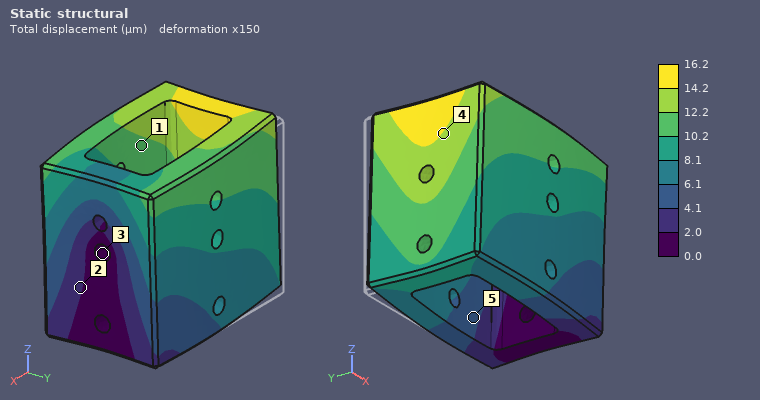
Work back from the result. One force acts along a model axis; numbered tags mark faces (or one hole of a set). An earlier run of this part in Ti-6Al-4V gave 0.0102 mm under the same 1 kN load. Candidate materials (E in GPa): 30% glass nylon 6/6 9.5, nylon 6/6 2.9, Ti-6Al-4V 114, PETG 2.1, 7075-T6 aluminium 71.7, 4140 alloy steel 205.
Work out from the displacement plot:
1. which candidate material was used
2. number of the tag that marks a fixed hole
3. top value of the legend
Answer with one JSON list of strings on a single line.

["7075-T6 aluminium", "3", "16.2 µm"]
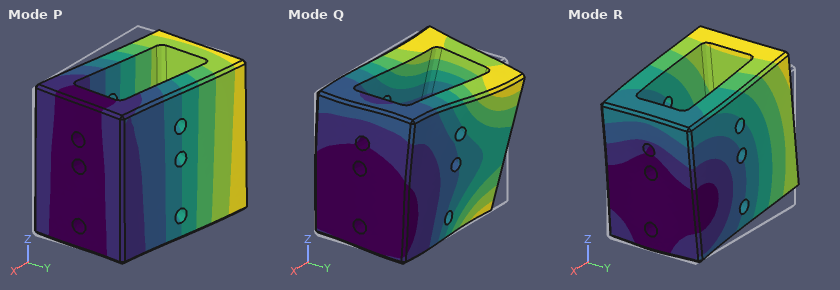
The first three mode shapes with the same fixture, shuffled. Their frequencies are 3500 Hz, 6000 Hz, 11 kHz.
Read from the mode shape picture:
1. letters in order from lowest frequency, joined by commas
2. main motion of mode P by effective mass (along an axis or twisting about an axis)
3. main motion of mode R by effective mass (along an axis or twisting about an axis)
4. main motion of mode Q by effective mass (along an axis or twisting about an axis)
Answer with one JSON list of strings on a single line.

["P, R, Q", "along Y", "along Z", "twisting about X"]
